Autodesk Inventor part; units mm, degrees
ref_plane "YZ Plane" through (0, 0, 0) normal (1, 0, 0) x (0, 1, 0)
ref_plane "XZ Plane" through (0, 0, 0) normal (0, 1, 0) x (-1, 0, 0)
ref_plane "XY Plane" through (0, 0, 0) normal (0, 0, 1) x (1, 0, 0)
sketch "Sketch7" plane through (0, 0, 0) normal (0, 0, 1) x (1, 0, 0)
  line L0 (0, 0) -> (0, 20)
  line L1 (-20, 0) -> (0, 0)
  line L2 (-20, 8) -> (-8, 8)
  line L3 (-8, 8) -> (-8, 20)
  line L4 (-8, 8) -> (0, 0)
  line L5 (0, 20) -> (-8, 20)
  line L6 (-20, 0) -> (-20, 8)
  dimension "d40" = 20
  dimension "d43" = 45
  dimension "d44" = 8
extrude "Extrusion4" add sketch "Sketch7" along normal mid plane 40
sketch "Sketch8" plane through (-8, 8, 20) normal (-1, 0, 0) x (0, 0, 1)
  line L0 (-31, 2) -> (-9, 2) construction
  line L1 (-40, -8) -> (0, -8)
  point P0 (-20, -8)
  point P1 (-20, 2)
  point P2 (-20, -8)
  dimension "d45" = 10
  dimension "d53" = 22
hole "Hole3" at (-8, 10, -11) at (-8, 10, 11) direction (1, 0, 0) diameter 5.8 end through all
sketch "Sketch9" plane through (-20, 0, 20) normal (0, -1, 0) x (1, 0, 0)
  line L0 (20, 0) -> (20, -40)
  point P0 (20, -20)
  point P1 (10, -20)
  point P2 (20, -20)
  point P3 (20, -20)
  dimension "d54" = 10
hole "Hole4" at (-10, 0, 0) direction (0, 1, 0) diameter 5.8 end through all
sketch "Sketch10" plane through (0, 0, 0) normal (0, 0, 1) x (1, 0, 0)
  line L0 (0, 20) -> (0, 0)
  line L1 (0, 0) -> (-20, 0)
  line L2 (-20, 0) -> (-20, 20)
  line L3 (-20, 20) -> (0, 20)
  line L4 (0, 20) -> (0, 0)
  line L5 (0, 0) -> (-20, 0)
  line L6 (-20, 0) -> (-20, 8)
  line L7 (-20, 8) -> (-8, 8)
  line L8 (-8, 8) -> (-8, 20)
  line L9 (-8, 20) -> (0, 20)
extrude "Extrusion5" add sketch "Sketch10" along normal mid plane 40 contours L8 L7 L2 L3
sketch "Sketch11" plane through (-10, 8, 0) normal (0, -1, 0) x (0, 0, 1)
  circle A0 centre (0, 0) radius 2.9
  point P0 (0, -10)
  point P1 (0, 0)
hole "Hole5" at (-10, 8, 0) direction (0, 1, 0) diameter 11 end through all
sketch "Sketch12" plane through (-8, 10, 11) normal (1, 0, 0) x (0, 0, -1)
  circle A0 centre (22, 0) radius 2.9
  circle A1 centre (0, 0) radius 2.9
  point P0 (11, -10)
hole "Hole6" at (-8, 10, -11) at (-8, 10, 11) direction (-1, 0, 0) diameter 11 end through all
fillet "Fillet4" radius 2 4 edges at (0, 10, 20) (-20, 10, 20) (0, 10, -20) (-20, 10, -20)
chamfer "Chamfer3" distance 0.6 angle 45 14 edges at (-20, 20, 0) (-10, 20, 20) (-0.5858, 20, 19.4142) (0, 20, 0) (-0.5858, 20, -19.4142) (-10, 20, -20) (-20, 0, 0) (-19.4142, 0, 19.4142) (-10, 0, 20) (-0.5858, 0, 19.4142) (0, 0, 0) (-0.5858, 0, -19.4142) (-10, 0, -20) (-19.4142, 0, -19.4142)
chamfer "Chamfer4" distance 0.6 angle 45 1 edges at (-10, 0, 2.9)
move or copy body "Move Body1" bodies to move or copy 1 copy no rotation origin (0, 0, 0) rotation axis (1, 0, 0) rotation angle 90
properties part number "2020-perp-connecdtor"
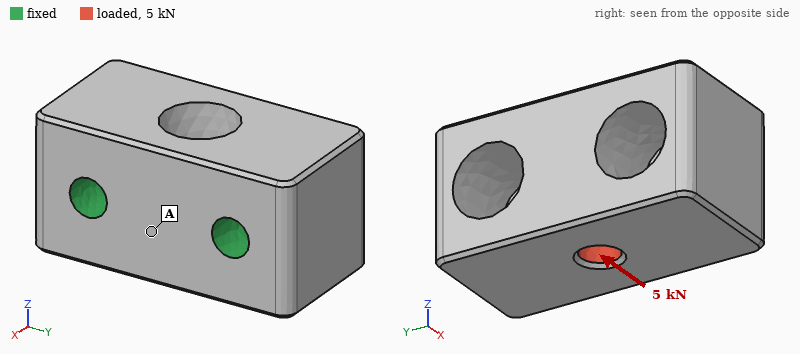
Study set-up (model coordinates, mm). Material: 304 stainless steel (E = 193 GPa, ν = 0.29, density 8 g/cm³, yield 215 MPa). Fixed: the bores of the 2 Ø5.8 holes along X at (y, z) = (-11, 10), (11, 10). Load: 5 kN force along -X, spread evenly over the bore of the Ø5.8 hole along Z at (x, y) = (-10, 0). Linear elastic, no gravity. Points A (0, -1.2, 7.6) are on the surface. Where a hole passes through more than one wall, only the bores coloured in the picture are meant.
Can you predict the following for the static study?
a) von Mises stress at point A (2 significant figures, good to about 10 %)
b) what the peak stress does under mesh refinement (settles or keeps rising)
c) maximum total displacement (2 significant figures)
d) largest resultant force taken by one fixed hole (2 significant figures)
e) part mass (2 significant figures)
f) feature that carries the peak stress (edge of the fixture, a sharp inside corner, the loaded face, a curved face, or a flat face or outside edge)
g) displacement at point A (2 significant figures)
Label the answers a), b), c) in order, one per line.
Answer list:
a) 25 MPa
b) keeps rising
c) 6.1 µm
d) 2.5 kN
e) 95 g
f) edge of the fixture
g) 2.5 µm
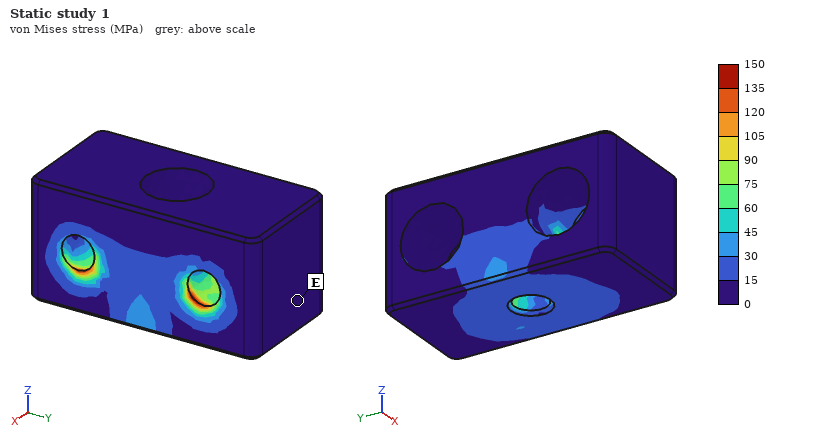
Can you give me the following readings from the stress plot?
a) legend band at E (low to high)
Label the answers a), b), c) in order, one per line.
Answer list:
a) 0 to 15 MPa
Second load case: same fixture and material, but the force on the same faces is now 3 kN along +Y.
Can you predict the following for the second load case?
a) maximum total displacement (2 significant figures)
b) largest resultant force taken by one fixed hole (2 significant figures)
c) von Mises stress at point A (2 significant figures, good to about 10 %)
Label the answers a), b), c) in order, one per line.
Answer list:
a) 2.4 µm
b) 1.7 kN
c) 8.1 MPa
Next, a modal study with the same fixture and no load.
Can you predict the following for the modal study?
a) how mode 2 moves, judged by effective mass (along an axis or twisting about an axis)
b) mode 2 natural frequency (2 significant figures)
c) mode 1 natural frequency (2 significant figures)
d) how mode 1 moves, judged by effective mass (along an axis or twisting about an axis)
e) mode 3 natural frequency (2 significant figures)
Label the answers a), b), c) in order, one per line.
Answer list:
a) along Y
b) 23 kHz
c) 17 kHz
d) along Z
e) 26 kHz
